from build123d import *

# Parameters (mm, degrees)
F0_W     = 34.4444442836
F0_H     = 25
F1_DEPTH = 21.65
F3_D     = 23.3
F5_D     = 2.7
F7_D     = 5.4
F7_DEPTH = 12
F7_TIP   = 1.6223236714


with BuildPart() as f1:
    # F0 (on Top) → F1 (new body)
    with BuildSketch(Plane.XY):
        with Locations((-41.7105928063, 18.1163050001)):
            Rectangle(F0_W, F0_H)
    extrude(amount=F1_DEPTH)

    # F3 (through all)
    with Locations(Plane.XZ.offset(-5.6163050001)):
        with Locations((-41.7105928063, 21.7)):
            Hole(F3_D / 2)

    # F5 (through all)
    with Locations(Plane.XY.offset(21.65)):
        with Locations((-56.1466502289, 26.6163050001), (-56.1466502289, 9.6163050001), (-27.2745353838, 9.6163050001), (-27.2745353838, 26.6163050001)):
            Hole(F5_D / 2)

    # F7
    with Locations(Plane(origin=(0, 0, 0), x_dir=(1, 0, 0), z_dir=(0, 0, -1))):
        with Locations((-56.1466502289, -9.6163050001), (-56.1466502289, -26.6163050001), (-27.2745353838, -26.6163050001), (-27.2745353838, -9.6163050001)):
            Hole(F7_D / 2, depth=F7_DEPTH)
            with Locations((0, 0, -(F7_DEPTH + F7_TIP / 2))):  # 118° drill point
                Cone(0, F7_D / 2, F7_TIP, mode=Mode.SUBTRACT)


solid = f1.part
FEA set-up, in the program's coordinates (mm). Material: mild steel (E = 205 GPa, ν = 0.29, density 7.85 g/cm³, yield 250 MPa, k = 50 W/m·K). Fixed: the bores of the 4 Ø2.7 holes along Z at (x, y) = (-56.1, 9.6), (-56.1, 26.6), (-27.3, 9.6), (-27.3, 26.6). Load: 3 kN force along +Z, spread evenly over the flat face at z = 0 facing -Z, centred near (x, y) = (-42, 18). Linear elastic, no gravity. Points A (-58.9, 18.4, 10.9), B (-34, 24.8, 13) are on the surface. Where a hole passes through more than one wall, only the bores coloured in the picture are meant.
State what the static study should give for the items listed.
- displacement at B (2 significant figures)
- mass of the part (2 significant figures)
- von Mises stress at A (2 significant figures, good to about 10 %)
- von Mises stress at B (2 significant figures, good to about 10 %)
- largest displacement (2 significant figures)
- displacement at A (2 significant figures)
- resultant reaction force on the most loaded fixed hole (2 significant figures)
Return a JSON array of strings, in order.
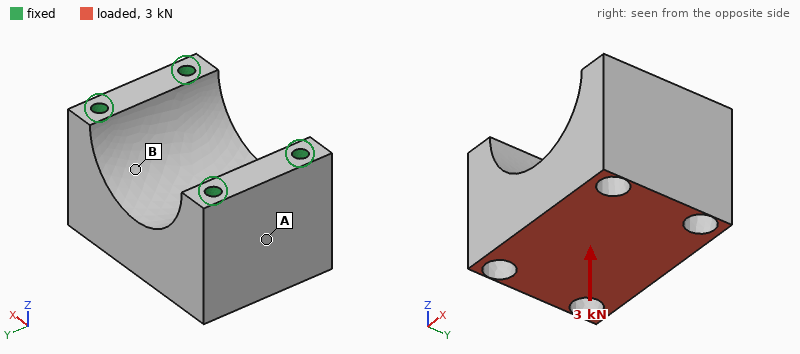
["0.67 µm", "94 g", "2.7 MPa", "9.2 MPa", "1.1 µm", "0.44 µm", "830 N"]
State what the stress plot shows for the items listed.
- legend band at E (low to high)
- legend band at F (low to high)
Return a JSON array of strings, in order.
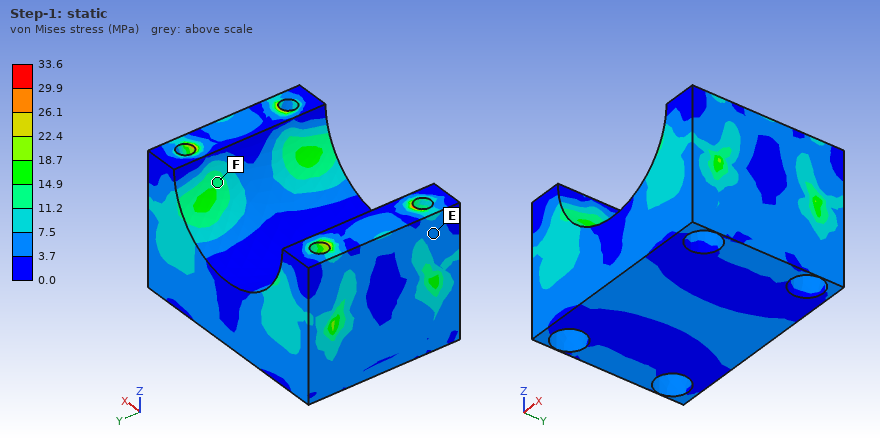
["3.7 to 7.5 MPa", "11.2 to 14.9 MPa"]
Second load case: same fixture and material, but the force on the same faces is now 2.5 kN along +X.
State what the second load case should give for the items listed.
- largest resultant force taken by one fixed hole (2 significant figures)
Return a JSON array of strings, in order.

["900 N"]
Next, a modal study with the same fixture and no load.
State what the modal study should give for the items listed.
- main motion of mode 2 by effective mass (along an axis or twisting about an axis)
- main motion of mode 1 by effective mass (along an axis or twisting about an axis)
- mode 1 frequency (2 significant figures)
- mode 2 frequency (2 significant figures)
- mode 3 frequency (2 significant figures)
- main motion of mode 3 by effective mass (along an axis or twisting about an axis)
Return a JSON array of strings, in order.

["along X", "along Y", "24 kHz", "28 kHz", "35 kHz", "twisting about Z"]
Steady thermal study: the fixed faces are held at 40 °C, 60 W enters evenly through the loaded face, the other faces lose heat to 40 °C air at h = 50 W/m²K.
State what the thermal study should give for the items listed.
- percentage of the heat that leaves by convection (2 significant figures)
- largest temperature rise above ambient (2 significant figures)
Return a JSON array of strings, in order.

["7.4 %", "45 K"]
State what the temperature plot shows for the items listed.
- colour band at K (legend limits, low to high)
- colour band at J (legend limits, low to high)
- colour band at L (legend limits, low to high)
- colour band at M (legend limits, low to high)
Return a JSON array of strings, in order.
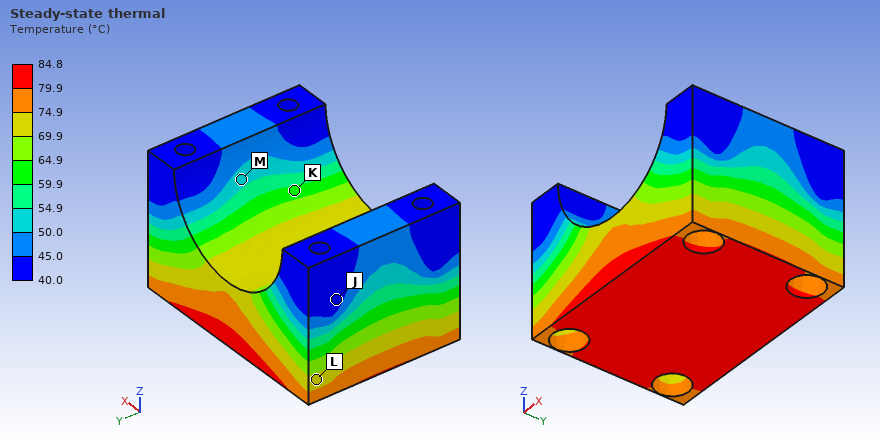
["59.9 to 64.9 °C", "40.0 to 45.0 °C", "69.9 to 74.9 °C", "50.0 to 54.9 °C"]
